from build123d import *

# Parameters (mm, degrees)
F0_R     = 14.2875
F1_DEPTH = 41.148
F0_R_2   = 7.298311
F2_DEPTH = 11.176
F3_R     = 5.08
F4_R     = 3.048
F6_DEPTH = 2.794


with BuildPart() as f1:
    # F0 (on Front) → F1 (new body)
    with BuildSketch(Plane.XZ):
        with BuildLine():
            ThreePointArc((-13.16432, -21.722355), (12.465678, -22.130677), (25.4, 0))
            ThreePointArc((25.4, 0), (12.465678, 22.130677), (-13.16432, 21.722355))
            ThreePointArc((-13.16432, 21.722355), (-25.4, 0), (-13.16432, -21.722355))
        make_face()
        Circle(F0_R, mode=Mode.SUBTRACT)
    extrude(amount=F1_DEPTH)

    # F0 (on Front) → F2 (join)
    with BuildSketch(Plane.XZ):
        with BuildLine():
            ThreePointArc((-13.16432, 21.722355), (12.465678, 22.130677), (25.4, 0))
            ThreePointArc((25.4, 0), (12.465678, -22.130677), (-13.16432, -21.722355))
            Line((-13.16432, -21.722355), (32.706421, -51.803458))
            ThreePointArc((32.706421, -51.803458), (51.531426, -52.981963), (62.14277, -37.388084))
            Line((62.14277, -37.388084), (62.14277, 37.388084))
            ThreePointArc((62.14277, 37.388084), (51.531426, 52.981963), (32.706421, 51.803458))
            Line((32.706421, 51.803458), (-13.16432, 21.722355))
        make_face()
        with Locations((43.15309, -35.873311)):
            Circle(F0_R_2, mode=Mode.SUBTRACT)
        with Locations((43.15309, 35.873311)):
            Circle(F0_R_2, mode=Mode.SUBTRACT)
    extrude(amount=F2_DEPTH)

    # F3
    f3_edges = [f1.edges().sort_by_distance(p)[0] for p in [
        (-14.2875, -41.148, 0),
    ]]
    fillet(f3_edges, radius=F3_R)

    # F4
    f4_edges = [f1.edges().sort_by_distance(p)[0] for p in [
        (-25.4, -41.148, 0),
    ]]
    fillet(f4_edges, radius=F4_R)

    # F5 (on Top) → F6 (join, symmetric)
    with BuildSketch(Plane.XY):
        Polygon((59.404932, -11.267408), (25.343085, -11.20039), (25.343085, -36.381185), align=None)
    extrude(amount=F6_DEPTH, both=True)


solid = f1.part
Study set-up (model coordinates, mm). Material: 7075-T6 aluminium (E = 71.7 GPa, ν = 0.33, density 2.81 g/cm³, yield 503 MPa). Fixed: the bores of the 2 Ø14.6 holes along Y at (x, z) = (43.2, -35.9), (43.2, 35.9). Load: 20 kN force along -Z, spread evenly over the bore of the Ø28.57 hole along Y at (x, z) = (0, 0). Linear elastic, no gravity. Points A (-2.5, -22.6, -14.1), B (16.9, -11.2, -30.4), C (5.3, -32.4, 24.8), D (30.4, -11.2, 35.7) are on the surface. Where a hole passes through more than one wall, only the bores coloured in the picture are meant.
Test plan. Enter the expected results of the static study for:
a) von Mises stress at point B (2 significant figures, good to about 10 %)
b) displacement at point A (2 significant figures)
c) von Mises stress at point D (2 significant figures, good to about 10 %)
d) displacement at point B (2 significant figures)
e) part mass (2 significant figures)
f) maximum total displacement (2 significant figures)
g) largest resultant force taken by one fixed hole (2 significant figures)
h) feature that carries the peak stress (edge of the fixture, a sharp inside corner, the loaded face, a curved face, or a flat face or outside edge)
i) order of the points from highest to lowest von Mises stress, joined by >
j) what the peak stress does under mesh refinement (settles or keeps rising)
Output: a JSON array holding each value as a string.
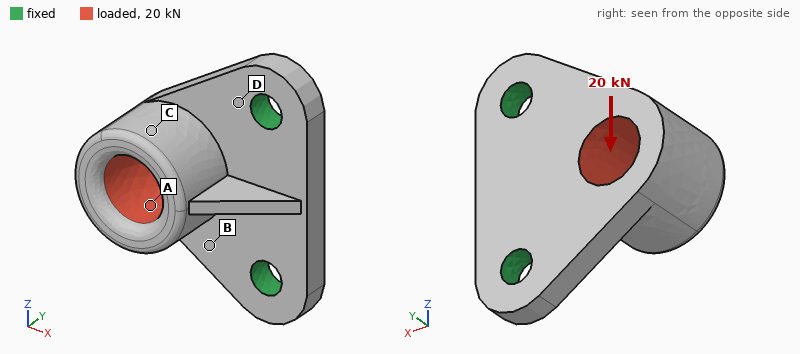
["71 MPa", "0.087 mm", "36 MPa", "0.041 mm", "300 g", "0.14 mm", "15 kN", "a sharp inside corner", "B > D > A > C", "keeps rising"]
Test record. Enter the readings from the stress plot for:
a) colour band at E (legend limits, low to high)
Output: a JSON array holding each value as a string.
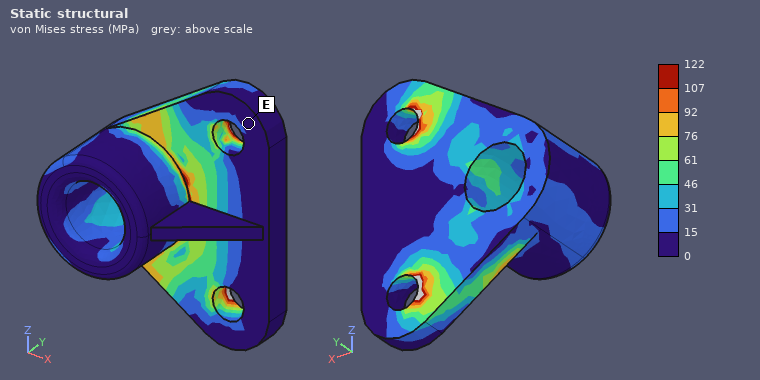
["0 to 15 MPa"]
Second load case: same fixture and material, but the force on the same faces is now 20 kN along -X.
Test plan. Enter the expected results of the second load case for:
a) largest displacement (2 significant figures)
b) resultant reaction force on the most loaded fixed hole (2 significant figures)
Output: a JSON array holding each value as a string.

["0.61 mm", "11 kN"]
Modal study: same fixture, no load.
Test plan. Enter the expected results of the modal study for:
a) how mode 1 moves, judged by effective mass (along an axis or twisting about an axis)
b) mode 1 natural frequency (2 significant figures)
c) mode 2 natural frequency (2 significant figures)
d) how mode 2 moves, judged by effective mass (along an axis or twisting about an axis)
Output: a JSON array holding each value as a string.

["along Y", "1700 Hz", "4700 Hz", "along Z"]
